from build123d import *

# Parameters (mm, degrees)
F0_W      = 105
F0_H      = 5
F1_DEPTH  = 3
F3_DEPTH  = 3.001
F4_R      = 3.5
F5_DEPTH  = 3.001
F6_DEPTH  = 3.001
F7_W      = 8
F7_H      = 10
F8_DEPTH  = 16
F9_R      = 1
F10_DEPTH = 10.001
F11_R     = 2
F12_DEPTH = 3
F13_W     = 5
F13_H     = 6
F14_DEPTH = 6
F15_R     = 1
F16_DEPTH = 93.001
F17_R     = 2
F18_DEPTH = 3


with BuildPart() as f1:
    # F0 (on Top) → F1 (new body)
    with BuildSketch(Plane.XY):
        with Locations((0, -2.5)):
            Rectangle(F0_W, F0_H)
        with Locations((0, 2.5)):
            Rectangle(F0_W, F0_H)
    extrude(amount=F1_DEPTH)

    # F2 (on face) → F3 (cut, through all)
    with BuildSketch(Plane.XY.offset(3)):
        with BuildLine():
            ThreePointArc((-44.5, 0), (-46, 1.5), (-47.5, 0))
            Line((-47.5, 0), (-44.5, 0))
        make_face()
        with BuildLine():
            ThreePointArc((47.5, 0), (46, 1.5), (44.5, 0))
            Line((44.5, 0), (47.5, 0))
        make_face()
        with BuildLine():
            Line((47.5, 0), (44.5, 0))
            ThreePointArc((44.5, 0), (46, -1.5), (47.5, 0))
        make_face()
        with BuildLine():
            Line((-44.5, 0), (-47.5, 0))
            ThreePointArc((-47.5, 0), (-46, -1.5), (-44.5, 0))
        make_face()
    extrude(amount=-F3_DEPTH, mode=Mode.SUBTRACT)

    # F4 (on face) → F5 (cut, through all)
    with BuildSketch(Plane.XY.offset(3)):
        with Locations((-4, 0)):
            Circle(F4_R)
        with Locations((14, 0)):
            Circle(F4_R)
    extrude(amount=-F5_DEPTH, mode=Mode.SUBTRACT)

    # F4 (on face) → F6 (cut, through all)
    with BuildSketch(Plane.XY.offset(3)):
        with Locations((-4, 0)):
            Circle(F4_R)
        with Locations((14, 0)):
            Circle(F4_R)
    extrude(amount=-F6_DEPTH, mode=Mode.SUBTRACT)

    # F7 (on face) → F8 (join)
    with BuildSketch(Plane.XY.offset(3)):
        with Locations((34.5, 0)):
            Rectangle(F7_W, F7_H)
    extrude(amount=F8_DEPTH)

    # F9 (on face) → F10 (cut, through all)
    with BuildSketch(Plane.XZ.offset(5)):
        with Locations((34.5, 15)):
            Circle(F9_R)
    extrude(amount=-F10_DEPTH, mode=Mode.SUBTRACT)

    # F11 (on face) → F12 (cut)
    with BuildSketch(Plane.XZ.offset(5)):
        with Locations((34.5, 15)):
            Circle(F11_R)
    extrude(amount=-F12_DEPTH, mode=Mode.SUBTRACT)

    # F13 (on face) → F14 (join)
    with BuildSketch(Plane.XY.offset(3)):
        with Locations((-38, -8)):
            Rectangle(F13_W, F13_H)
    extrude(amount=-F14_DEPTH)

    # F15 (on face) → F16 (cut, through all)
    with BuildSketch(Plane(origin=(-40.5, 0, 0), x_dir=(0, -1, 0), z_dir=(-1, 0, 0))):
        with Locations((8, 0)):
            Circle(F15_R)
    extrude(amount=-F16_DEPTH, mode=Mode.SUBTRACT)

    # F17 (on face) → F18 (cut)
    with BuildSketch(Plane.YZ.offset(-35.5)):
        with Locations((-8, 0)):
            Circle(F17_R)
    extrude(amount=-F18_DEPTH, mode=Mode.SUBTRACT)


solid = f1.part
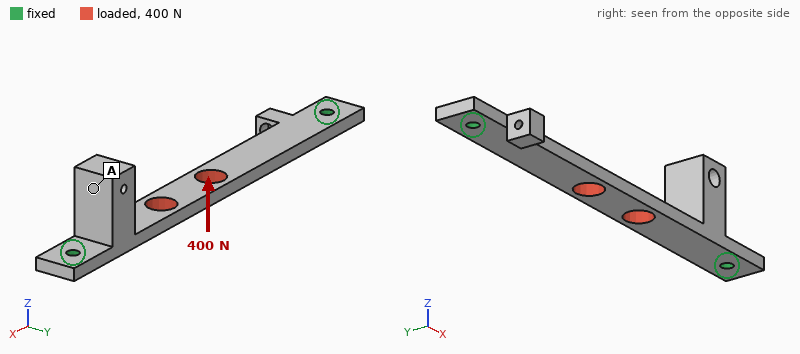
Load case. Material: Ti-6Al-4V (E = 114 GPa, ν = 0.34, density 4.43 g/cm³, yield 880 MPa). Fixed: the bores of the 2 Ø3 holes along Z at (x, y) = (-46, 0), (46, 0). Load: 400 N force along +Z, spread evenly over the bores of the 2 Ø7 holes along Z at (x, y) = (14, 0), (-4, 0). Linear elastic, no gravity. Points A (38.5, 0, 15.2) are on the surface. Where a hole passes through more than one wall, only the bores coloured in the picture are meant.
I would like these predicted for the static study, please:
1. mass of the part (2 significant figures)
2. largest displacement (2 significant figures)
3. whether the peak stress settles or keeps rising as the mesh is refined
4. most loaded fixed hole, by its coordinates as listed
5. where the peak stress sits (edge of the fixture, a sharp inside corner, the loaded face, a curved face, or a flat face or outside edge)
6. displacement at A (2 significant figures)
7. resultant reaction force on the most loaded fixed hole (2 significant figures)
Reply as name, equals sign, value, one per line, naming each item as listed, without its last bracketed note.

mass of the part = 19 g
largest displacement = 0.64 mm
whether the peak stress settles or keeps rising as the mesh is refined = keeps rising
most loaded fixed hole, by its coordinates as listed = (46, 0)
where the peak stress sits = edge of the fixture
displacement at A = 0.22 mm
resultant reaction force on the most loaded fixed hole = 250 N
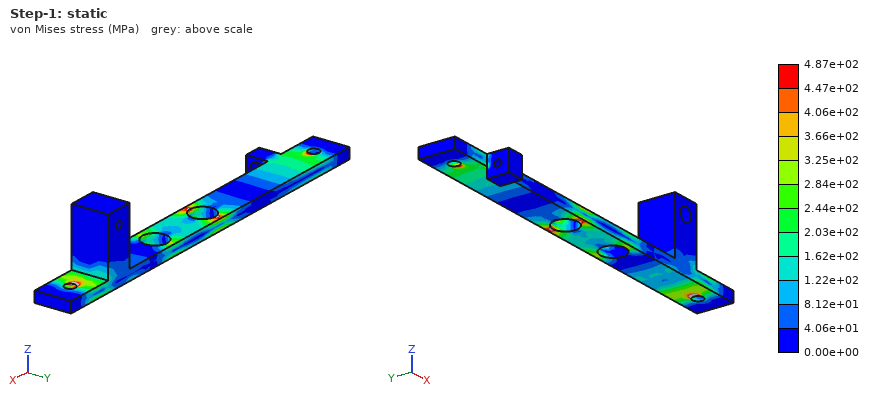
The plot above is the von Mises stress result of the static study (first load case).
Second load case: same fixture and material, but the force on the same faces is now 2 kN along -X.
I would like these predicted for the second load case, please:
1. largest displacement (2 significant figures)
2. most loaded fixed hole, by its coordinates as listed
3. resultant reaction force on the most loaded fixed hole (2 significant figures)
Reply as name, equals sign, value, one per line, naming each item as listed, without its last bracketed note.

largest displacement = 16 µm
most loaded fixed hole, by its coordinates as listed = (46, 0)
resultant reaction force on the most loaded fixed hole = 1.1 kN
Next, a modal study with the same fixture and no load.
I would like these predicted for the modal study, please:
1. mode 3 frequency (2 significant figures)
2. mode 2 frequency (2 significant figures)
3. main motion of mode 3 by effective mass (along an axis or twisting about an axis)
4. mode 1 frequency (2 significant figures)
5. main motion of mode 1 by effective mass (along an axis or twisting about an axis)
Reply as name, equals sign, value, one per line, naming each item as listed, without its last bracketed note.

mode 3 frequency = 4100 Hz
mode 2 frequency = 3900 Hz
main motion of mode 3 by effective mass = along Y
mode 1 frequency = 1800 Hz
main motion of mode 1 by effective mass = along Z
